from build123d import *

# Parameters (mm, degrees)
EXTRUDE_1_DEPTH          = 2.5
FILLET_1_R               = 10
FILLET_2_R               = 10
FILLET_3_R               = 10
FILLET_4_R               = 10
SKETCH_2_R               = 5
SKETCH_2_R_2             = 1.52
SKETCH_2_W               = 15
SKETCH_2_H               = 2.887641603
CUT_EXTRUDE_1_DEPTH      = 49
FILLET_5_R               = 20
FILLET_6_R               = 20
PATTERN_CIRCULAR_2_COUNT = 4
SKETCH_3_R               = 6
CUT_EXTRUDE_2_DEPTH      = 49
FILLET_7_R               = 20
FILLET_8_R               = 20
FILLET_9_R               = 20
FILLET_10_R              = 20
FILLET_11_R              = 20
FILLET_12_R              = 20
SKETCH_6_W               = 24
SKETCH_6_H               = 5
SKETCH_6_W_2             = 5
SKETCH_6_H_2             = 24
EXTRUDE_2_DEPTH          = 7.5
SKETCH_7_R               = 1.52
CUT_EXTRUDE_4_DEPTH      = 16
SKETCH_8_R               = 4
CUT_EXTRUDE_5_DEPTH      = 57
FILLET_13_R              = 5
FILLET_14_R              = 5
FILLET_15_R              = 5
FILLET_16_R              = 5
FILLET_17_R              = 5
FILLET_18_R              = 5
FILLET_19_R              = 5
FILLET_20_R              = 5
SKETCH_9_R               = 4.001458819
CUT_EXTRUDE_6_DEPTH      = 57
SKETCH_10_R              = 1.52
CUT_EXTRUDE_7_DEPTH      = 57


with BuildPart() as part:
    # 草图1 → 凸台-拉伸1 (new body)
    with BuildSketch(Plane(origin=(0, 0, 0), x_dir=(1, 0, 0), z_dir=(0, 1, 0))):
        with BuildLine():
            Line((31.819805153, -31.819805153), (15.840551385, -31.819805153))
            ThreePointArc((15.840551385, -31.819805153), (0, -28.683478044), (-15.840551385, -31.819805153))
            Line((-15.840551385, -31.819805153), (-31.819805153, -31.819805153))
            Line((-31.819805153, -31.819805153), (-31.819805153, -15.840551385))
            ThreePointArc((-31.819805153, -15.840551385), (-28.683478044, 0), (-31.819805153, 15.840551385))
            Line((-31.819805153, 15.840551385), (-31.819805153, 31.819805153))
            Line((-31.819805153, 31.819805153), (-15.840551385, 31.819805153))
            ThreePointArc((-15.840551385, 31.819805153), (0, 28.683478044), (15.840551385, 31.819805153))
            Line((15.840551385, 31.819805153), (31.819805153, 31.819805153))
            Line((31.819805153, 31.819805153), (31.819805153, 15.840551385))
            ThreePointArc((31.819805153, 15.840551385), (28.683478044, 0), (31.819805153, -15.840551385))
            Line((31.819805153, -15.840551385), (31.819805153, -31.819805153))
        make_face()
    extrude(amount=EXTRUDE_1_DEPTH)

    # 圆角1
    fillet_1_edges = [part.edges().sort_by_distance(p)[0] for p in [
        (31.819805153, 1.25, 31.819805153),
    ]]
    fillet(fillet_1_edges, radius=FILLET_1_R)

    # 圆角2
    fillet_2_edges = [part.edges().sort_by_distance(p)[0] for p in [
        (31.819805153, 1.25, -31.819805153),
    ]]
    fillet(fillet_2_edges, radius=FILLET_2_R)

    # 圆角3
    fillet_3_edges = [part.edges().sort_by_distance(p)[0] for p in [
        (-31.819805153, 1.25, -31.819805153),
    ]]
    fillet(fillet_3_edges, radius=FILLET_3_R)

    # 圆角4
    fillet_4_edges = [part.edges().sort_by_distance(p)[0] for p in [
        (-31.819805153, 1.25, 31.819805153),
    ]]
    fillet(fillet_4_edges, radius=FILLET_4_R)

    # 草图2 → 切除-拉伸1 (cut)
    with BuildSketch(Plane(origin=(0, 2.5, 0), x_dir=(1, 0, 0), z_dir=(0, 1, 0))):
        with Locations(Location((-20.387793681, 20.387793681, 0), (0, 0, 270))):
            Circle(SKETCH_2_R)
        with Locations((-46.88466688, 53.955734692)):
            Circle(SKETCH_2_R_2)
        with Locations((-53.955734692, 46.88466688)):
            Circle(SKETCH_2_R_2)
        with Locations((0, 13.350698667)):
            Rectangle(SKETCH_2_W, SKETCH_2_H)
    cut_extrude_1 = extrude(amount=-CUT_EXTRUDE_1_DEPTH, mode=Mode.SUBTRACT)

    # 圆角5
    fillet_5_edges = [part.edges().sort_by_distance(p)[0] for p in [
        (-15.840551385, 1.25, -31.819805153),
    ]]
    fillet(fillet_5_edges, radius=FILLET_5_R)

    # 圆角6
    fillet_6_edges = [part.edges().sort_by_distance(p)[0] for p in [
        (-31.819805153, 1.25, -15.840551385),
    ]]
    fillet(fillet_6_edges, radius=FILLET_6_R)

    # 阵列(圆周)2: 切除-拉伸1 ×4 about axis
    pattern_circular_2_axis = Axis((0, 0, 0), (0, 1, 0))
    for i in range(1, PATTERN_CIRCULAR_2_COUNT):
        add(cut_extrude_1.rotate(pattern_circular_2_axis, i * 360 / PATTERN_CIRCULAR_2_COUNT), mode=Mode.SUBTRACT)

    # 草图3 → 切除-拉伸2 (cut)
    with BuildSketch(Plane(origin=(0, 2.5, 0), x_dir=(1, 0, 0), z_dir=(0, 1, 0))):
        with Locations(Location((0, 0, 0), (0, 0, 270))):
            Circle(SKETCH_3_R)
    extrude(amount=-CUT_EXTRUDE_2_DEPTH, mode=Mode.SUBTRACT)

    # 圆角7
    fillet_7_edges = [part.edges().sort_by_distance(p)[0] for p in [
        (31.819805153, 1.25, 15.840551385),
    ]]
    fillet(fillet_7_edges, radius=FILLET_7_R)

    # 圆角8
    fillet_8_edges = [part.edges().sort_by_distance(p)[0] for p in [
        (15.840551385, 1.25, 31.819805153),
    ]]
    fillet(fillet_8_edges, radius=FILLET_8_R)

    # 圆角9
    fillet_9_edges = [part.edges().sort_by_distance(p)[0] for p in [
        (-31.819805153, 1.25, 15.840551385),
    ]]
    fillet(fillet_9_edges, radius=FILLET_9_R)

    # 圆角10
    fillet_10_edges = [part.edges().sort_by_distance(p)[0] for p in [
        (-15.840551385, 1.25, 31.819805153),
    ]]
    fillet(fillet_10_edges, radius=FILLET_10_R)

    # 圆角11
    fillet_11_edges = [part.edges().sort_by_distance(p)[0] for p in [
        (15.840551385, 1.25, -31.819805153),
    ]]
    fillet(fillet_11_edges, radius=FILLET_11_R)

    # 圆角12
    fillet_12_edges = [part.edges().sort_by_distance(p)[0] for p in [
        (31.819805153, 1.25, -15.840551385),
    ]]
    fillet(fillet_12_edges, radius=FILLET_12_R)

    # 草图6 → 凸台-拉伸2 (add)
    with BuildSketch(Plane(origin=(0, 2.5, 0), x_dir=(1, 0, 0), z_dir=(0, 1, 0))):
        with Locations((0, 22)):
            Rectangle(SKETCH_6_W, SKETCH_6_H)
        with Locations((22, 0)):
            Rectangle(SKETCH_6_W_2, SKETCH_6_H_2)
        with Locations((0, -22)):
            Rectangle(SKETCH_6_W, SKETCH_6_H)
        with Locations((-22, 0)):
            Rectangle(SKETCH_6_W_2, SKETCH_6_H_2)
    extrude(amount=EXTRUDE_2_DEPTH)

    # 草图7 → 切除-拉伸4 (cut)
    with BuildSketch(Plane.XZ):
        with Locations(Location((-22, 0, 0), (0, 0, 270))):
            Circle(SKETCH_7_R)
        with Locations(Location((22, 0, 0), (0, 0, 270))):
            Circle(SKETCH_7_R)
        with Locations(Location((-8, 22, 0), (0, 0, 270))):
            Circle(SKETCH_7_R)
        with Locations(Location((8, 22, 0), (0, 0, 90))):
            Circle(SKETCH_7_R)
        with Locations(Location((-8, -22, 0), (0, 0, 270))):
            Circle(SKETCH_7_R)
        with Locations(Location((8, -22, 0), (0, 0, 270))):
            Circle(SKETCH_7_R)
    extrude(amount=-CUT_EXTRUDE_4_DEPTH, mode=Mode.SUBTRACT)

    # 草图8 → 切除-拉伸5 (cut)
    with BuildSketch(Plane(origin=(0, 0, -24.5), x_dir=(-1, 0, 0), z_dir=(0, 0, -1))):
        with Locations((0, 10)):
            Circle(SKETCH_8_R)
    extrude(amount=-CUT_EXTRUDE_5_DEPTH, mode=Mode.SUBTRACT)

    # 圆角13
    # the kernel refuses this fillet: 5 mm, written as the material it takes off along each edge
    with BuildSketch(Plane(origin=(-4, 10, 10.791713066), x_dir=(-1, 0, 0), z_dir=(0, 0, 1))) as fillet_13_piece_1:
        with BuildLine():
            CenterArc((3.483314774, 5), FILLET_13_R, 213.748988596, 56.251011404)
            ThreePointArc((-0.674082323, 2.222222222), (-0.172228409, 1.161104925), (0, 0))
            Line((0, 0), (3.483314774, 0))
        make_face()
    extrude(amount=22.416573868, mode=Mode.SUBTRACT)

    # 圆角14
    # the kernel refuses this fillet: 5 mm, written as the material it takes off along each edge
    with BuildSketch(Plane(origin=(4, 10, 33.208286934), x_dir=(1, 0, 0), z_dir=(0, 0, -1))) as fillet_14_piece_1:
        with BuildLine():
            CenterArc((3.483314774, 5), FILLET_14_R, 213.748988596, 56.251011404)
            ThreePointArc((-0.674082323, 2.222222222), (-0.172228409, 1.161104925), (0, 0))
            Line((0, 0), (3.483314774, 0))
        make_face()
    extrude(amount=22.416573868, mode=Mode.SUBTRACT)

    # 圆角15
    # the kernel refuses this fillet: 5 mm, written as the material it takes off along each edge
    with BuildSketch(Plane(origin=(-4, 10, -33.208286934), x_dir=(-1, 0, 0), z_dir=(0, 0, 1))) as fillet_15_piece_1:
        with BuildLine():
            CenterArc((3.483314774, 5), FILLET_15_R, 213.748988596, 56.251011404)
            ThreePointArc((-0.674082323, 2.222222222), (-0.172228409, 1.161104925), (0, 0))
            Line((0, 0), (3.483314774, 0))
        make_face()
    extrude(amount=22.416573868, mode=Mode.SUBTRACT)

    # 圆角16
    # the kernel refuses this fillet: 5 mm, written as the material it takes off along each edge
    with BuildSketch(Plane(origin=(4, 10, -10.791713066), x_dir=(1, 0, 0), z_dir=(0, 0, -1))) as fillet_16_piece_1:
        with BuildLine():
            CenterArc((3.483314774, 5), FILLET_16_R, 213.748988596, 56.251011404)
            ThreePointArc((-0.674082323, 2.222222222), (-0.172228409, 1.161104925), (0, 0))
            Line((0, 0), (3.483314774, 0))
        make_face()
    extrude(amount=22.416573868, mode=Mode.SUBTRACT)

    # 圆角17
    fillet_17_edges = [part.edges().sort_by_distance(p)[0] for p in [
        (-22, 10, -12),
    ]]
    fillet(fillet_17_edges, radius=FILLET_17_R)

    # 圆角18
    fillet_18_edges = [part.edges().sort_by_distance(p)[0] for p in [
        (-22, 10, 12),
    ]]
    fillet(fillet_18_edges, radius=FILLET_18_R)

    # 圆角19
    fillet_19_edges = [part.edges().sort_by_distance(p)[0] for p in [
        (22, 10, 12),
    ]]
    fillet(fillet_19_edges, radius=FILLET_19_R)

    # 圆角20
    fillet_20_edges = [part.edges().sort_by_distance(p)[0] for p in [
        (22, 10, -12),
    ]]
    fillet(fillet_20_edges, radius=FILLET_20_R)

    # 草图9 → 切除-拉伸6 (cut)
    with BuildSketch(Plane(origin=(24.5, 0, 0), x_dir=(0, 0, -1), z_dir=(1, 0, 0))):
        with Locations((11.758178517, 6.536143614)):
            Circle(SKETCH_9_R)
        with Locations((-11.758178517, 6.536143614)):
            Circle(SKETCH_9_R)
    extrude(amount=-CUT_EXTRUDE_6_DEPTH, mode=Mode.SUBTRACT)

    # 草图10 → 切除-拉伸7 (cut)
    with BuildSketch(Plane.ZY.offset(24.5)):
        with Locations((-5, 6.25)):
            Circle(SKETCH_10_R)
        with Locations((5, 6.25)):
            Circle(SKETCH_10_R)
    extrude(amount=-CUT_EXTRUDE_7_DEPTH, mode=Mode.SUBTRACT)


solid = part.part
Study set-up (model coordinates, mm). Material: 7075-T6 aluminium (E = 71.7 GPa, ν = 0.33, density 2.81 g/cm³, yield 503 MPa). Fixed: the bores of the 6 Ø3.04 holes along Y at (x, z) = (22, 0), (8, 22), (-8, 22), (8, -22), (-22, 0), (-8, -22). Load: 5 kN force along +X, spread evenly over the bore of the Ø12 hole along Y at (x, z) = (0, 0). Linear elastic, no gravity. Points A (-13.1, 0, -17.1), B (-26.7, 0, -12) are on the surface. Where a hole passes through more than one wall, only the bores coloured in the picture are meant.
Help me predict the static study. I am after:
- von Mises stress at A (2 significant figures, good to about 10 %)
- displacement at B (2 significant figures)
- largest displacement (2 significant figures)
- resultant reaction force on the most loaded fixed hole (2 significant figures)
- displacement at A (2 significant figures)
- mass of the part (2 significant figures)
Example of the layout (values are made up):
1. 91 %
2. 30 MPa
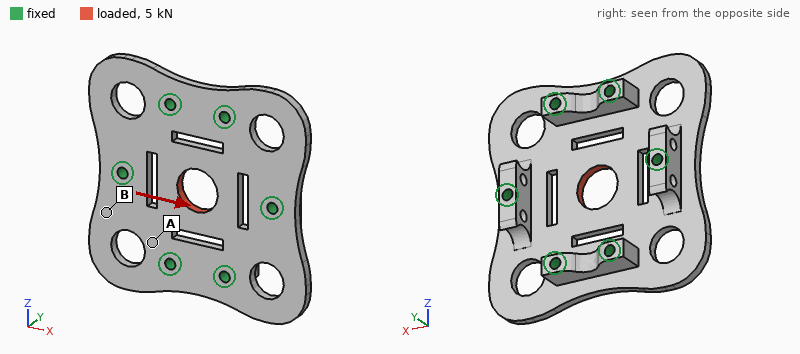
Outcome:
1. 52 MPa
2. 8.6 µm
3. 36 µm
4. 1.2 kN
5. 6.7 µm
6. 28 g
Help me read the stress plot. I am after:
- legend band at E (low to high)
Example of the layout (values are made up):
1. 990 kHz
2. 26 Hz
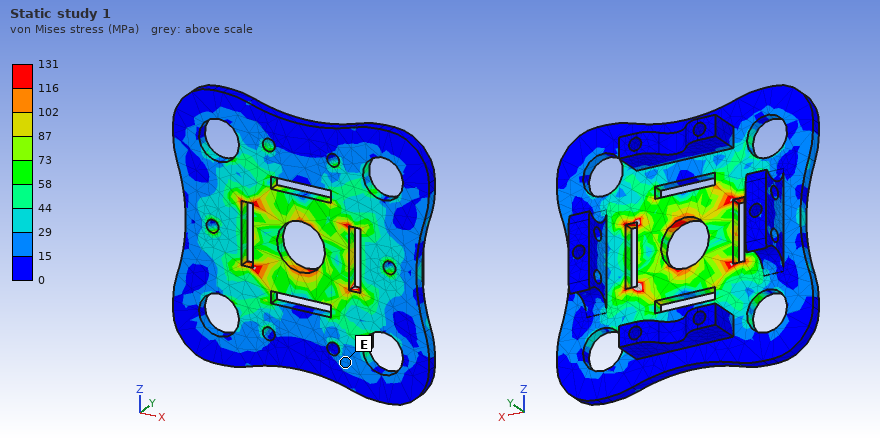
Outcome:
1. 15 to 29 MPa
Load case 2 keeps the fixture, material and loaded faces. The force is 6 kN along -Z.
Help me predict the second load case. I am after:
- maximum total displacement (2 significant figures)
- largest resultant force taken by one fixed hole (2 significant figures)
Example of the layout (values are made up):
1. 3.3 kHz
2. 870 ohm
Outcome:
1. 38 µm
2. 1.2 kN
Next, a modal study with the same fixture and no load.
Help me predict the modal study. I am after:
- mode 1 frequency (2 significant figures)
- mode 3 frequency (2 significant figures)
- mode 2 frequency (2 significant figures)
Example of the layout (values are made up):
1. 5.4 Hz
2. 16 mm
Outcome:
1. 6800 Hz
2. 6900 Hz
3. 6900 Hz
